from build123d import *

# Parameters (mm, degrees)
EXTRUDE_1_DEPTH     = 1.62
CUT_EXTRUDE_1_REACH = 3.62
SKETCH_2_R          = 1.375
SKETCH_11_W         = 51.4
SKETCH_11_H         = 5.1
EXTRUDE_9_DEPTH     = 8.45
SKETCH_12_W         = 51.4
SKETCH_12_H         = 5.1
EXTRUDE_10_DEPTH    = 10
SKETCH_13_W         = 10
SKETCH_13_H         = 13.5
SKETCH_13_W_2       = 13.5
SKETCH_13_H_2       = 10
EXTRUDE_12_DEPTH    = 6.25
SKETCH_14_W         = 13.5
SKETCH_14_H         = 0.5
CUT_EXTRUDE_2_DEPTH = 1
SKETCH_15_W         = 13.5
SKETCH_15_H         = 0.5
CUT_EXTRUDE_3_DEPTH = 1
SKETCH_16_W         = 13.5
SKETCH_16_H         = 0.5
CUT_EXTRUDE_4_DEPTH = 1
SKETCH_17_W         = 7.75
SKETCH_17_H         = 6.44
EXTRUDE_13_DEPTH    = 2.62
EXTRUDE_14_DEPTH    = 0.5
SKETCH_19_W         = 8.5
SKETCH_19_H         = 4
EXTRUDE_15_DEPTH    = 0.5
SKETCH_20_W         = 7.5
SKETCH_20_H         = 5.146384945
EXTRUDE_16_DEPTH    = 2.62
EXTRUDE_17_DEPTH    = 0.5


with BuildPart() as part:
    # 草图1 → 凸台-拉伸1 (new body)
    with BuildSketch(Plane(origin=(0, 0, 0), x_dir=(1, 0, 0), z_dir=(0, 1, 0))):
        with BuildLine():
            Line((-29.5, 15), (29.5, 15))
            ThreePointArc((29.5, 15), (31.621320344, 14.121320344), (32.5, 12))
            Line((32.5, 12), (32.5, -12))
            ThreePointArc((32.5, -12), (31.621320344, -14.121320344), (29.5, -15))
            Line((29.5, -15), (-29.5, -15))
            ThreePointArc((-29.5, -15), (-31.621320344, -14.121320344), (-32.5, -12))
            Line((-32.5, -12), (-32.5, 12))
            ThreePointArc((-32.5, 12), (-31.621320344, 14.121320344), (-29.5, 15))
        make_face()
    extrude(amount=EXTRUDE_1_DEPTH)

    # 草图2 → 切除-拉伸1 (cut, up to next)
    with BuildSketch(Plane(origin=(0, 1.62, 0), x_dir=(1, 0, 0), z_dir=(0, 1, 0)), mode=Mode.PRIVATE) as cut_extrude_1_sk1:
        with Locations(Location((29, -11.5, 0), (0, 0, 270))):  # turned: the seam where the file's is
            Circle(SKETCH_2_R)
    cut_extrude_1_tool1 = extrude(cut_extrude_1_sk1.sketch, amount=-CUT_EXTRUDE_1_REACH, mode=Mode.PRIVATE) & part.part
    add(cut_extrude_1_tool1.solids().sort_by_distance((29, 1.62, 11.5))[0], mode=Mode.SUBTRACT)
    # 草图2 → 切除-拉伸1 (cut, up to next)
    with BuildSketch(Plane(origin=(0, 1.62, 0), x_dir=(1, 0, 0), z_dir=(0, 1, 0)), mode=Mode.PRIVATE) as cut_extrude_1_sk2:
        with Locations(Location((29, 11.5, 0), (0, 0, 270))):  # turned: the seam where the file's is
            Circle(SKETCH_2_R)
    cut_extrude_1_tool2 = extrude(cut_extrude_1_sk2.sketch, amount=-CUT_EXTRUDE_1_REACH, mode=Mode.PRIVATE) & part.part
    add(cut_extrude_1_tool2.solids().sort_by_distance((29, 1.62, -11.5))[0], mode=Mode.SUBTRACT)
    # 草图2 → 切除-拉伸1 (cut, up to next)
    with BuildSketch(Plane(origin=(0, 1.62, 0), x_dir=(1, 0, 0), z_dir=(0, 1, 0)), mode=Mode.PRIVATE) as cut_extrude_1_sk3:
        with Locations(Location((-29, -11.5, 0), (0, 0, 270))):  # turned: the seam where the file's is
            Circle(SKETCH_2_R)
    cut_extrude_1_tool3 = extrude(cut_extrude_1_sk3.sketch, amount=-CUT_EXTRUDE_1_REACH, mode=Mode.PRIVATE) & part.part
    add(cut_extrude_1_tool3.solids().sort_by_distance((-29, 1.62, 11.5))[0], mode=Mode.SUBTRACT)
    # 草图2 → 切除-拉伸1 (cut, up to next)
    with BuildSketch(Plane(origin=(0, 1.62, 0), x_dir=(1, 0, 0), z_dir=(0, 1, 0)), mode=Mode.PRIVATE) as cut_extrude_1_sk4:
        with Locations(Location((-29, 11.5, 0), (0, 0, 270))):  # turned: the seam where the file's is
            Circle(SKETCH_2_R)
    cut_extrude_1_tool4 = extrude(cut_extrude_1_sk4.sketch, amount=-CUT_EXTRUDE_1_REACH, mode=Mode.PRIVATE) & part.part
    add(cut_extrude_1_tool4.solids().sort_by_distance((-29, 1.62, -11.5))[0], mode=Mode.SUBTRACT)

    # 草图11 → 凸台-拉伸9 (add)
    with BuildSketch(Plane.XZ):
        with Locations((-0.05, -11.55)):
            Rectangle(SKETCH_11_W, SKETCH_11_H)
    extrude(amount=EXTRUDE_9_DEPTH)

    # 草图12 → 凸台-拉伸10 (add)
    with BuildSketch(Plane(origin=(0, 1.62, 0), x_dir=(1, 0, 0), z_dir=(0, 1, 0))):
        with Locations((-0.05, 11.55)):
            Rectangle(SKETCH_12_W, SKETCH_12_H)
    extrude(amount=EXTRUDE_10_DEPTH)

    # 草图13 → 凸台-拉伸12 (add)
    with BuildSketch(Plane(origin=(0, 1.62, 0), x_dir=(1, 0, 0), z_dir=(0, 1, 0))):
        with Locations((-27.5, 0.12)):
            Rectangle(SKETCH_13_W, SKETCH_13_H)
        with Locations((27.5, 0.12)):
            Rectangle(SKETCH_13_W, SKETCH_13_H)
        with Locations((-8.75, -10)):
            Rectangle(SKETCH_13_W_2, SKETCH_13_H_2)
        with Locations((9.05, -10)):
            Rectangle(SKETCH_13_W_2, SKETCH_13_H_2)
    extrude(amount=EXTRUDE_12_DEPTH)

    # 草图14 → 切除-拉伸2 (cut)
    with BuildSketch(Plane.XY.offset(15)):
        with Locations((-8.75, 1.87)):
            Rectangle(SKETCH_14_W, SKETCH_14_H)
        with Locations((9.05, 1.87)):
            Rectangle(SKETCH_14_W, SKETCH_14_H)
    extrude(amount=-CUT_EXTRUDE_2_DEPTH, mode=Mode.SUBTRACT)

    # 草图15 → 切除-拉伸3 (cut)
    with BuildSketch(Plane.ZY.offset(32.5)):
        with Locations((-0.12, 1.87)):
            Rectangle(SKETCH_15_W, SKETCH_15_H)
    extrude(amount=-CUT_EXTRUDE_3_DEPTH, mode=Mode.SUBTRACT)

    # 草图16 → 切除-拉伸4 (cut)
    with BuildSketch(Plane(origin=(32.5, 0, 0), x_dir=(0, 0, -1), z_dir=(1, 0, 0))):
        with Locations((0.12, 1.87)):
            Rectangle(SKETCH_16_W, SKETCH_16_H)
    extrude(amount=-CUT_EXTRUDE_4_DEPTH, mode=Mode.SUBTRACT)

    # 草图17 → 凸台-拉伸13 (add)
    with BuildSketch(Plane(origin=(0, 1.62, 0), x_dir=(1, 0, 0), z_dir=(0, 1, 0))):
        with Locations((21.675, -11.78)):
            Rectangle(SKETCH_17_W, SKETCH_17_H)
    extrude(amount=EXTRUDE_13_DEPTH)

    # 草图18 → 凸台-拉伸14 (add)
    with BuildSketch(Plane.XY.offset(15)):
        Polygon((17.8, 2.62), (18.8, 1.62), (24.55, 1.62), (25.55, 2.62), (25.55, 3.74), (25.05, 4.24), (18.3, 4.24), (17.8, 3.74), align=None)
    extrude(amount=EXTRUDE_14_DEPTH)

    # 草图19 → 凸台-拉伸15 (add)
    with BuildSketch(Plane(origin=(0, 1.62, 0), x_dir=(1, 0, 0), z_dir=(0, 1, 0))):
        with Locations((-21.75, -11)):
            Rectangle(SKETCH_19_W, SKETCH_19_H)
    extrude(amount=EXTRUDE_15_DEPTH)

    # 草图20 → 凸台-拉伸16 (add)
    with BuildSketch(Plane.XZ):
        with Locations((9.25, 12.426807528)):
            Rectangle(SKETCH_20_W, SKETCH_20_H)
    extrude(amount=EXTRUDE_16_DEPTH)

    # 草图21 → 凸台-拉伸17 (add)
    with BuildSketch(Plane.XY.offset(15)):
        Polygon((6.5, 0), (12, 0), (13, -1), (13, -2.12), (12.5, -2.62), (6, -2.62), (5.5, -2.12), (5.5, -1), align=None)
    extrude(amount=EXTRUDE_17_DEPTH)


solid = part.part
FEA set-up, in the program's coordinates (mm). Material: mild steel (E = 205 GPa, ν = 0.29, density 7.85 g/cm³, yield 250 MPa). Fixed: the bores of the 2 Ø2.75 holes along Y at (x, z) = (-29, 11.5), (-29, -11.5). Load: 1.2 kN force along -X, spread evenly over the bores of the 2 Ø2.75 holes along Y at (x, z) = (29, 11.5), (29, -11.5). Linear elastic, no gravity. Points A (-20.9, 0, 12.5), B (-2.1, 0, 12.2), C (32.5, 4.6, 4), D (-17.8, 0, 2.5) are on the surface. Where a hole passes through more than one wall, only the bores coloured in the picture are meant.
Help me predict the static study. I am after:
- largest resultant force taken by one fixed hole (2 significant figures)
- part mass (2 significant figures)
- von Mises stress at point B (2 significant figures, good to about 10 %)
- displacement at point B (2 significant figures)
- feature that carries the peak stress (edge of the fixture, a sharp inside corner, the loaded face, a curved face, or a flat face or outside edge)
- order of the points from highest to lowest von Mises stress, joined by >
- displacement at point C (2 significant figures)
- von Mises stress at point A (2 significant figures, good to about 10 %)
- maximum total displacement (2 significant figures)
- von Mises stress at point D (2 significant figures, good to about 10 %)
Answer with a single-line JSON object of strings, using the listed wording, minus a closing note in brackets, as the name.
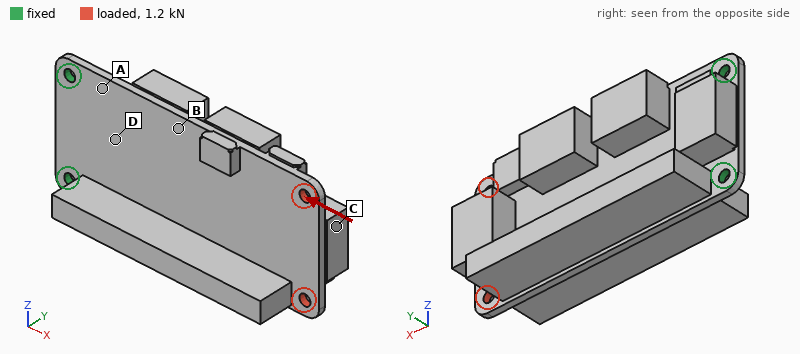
{"largest resultant force taken by one fixed hole": "610 N", "part mass": "91 g", "von Mises stress at point B": "26 MPa", "displacement at point B": "4.4 µm", "feature that carries the peak stress": "the loaded face", "order of the points from highest to lowest von Mises stress, joined by >": "A > B > D > C", "displacement at point C": "11 µm", "von Mises stress at point A": "36 MPa", "maximum total displacement": "14 µm", "von Mises stress at point D": "12 MPa"}
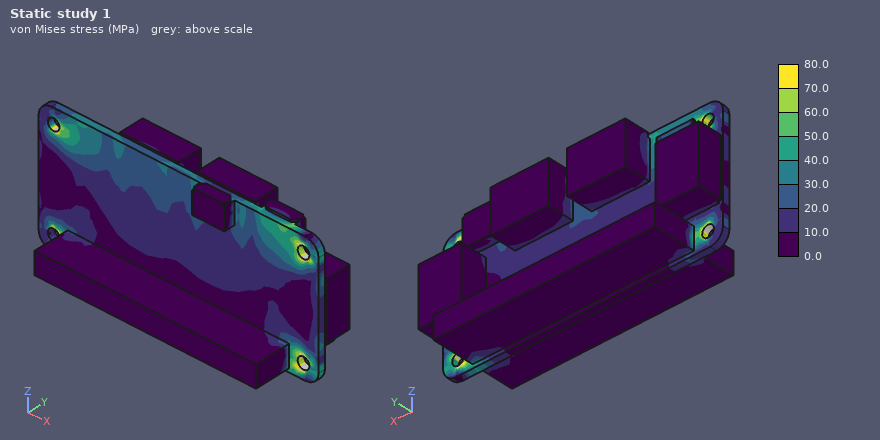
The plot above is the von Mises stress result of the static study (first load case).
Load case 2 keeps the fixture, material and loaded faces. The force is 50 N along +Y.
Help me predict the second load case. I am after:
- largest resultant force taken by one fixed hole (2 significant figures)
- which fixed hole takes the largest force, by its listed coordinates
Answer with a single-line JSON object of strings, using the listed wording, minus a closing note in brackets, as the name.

{"largest resultant force taken by one fixed hole": "34 N", "which fixed hole takes the largest force, by its listed coordinates": "(-29, 11.5)"}
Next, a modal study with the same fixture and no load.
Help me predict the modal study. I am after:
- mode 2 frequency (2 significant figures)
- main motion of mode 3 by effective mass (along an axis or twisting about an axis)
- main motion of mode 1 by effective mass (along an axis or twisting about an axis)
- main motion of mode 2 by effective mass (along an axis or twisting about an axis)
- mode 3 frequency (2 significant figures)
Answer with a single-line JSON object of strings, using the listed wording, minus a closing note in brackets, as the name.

{"mode 2 frequency": "1600 Hz", "main motion of mode 3 by effective mass": "along Z", "main motion of mode 1 by effective mass": "along Y", "main motion of mode 2 by effective mass": "twisting about X", "mode 3 frequency": "3500 Hz"}
